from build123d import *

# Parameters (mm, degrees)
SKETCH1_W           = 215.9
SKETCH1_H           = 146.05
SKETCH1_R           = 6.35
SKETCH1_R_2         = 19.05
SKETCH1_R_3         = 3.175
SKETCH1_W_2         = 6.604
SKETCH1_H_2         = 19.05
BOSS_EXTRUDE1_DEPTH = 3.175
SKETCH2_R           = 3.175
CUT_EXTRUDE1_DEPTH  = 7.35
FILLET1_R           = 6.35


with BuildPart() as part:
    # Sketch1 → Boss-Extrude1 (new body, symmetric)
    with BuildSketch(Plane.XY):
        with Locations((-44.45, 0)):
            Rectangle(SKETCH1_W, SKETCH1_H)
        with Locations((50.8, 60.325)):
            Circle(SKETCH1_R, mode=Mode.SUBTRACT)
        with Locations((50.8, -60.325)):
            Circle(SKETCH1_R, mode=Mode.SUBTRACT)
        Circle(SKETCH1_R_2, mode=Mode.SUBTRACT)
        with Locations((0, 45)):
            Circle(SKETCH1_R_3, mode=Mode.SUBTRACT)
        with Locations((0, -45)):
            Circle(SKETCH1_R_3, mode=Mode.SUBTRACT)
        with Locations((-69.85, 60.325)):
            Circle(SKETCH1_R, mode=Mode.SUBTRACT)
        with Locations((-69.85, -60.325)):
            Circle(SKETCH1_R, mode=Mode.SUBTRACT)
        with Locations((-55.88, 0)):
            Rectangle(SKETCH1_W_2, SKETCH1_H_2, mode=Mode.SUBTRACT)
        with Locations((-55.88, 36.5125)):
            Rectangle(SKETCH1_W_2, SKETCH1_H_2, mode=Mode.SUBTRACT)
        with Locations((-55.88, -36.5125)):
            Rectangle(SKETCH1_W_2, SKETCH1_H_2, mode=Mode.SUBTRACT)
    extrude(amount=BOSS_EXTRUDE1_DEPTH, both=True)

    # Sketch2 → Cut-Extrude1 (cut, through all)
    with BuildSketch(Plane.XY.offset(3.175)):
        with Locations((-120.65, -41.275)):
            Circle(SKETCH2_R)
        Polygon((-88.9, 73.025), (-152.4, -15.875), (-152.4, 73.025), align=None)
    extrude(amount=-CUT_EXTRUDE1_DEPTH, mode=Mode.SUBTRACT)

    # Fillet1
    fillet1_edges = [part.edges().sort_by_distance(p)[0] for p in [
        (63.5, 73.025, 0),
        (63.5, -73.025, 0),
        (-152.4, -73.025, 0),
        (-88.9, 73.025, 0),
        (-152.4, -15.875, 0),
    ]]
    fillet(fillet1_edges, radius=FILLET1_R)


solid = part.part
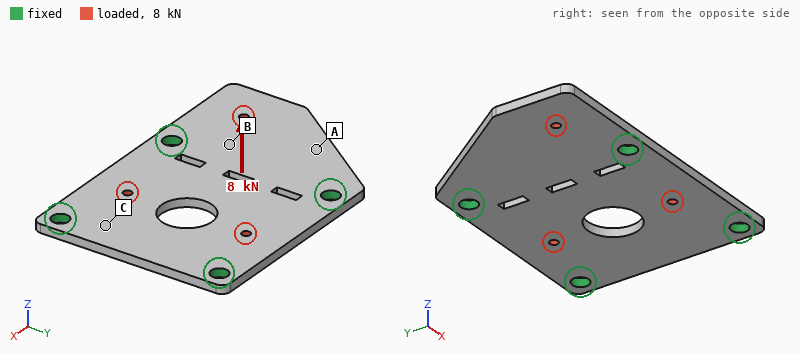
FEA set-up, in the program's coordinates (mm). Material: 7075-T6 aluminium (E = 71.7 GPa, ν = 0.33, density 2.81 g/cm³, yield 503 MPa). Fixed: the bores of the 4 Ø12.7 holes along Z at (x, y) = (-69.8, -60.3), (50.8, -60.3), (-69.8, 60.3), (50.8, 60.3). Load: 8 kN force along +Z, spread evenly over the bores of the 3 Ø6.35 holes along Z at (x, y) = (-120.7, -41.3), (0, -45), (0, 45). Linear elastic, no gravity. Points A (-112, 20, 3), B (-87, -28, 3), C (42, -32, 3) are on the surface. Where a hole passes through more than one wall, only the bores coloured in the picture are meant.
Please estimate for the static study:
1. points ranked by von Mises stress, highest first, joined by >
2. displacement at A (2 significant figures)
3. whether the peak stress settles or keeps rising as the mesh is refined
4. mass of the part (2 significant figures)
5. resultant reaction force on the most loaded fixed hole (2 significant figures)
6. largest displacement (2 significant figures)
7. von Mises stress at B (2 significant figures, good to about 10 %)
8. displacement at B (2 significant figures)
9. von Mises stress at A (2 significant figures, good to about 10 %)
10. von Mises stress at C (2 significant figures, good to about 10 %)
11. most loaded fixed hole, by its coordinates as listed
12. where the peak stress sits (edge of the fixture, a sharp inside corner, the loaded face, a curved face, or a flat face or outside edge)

B > A > C
0.45 mm
keeps rising
470 g
3.5 kN
1.6 mm
110 MPa
0.24 mm
62 MPa
30 MPa
(-69.8, -60.3)
edge of the fixture
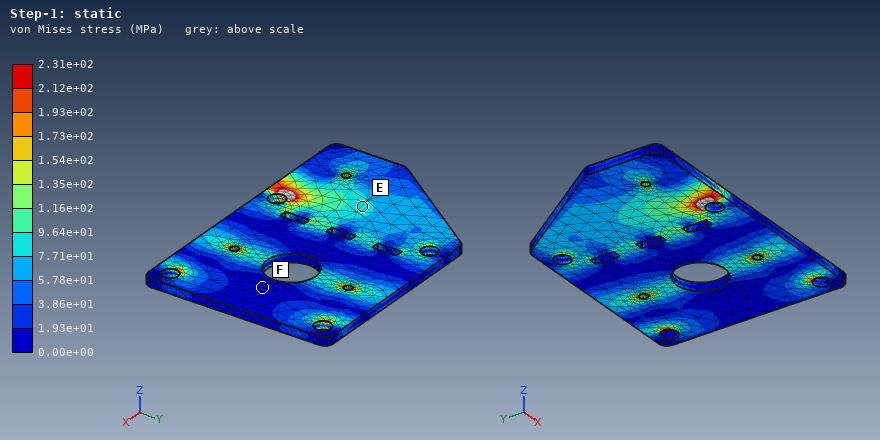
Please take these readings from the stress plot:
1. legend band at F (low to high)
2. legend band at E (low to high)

0.00e+00 to 1.93e+01 MPa
7.71e+01 to 9.64e+01 MPa
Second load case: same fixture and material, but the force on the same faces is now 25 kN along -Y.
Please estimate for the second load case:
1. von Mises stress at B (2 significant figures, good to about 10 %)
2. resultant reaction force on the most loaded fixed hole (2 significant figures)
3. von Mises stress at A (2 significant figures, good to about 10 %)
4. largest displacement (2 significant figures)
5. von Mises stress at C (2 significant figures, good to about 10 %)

17 MPa
7.9 kN
19 MPa
44 µm
17 MPa
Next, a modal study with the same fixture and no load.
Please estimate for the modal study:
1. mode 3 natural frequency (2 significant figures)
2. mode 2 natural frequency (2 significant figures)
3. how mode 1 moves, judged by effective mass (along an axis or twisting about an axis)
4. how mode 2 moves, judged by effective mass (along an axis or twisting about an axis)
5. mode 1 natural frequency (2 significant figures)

1900 Hz
1700 Hz
along Z
along Z
820 Hz
